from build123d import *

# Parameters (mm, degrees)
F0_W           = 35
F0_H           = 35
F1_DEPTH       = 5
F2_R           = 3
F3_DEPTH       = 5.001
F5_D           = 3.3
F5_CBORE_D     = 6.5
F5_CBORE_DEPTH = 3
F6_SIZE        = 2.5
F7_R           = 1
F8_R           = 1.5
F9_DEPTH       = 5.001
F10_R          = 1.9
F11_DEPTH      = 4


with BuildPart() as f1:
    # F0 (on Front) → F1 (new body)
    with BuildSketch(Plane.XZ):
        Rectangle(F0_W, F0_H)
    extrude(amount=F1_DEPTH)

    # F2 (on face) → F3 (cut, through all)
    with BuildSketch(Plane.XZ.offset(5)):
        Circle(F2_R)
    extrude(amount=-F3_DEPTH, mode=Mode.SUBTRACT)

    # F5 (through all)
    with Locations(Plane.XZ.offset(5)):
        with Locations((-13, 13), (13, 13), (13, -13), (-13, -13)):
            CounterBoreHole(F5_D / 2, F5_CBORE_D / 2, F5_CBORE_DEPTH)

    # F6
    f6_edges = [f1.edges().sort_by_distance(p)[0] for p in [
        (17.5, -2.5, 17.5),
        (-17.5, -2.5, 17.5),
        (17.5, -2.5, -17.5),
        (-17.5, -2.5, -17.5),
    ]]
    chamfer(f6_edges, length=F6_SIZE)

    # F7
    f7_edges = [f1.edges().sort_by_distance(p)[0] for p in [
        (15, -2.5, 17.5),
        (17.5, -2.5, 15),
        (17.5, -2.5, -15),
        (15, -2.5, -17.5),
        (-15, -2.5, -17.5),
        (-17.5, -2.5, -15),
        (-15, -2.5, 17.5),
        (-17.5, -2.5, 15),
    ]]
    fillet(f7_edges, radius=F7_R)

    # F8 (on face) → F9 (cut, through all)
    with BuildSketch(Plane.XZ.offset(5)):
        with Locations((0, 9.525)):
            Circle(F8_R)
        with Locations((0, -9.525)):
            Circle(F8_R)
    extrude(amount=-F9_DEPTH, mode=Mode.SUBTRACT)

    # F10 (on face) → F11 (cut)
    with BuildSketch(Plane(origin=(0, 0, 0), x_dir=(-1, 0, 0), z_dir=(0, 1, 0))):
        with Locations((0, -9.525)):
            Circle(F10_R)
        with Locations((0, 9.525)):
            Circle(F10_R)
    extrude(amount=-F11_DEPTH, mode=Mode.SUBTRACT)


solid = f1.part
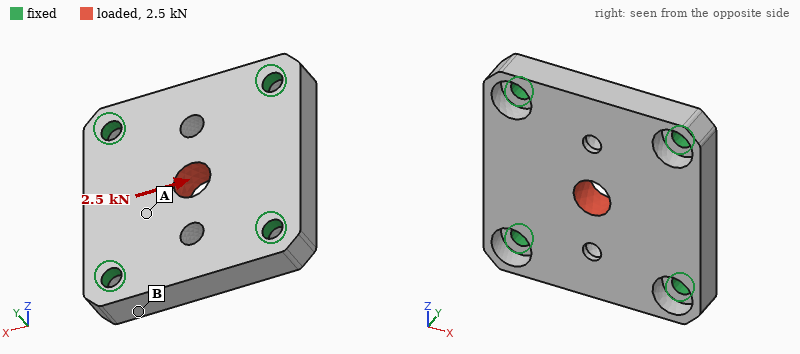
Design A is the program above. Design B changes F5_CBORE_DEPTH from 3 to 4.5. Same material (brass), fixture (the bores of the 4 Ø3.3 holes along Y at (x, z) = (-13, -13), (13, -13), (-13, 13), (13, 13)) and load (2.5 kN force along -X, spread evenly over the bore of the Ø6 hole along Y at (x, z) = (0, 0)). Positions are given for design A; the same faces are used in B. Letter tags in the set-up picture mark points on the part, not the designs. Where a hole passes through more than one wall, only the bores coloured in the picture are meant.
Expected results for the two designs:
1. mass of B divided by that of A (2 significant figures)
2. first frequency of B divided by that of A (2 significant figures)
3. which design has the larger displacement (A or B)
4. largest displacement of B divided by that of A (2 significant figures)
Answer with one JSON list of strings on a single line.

["0.97", "0.57", "B", "1.9"]
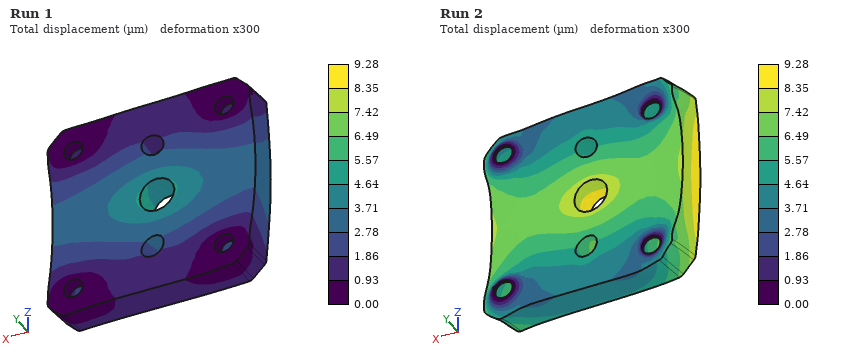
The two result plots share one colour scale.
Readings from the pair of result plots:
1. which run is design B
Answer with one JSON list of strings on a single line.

["Run 2"]
